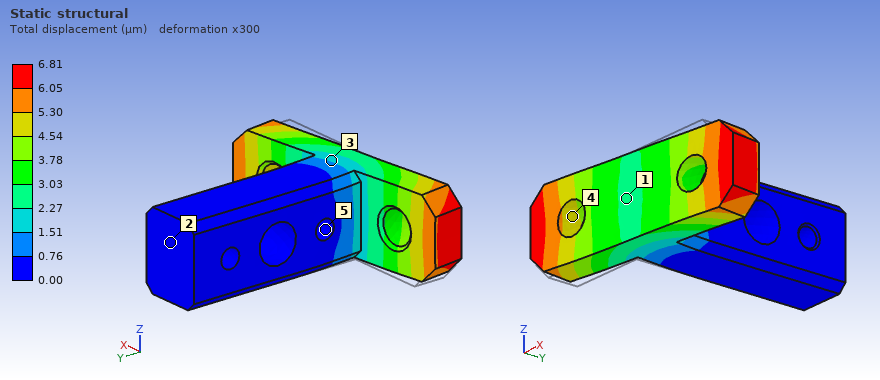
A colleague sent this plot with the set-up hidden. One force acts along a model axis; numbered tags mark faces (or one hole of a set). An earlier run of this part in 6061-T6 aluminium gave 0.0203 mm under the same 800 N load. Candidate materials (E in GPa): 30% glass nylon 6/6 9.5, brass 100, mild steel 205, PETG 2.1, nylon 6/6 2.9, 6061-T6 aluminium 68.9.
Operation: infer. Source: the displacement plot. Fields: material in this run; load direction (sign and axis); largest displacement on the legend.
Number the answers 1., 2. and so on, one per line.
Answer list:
1. mild steel
2. +X
3. 6.81 µm
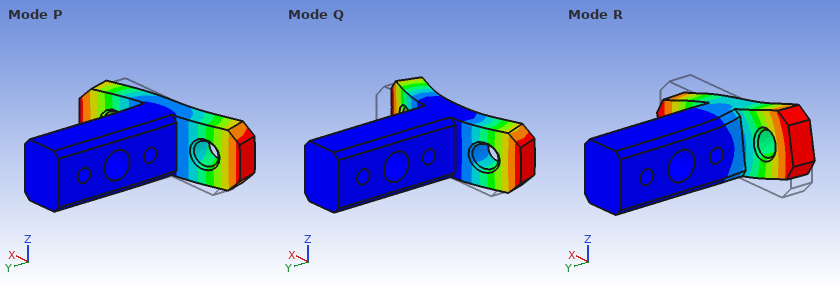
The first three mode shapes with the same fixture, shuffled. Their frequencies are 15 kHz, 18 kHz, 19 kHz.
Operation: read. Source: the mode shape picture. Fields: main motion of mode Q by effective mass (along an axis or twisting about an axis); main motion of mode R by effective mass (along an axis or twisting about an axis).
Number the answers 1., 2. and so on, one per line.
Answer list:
1. along Y
2. twisting about Y
